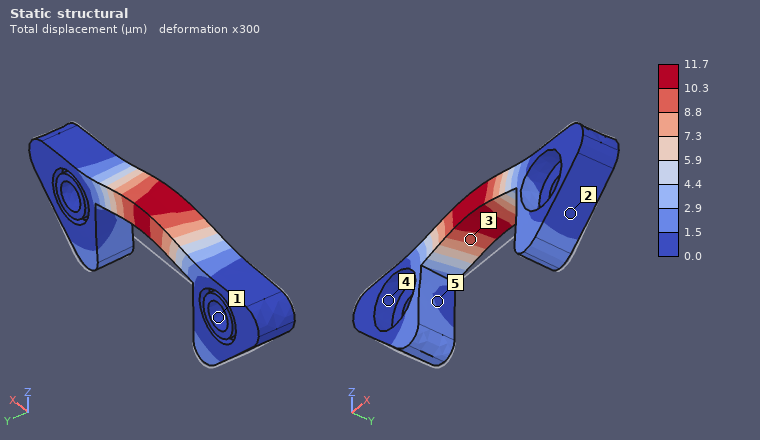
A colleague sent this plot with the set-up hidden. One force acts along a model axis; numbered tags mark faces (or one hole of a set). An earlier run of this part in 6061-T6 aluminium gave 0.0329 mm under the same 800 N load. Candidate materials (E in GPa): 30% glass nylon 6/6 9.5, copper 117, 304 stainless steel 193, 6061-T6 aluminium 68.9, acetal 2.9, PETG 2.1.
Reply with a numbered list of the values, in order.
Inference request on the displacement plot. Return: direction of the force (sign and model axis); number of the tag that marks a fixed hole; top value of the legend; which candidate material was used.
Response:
1. +Z
2. 1
3. 11.7 µm
4. 304 stainless steel
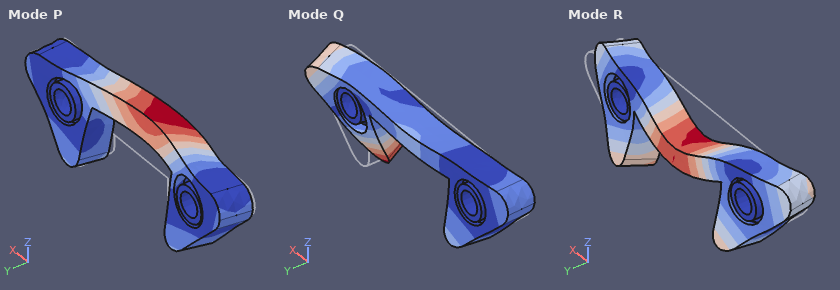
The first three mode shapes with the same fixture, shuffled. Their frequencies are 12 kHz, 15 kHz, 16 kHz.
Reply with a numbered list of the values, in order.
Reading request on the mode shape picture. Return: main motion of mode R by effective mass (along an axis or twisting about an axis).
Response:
1. along Z
